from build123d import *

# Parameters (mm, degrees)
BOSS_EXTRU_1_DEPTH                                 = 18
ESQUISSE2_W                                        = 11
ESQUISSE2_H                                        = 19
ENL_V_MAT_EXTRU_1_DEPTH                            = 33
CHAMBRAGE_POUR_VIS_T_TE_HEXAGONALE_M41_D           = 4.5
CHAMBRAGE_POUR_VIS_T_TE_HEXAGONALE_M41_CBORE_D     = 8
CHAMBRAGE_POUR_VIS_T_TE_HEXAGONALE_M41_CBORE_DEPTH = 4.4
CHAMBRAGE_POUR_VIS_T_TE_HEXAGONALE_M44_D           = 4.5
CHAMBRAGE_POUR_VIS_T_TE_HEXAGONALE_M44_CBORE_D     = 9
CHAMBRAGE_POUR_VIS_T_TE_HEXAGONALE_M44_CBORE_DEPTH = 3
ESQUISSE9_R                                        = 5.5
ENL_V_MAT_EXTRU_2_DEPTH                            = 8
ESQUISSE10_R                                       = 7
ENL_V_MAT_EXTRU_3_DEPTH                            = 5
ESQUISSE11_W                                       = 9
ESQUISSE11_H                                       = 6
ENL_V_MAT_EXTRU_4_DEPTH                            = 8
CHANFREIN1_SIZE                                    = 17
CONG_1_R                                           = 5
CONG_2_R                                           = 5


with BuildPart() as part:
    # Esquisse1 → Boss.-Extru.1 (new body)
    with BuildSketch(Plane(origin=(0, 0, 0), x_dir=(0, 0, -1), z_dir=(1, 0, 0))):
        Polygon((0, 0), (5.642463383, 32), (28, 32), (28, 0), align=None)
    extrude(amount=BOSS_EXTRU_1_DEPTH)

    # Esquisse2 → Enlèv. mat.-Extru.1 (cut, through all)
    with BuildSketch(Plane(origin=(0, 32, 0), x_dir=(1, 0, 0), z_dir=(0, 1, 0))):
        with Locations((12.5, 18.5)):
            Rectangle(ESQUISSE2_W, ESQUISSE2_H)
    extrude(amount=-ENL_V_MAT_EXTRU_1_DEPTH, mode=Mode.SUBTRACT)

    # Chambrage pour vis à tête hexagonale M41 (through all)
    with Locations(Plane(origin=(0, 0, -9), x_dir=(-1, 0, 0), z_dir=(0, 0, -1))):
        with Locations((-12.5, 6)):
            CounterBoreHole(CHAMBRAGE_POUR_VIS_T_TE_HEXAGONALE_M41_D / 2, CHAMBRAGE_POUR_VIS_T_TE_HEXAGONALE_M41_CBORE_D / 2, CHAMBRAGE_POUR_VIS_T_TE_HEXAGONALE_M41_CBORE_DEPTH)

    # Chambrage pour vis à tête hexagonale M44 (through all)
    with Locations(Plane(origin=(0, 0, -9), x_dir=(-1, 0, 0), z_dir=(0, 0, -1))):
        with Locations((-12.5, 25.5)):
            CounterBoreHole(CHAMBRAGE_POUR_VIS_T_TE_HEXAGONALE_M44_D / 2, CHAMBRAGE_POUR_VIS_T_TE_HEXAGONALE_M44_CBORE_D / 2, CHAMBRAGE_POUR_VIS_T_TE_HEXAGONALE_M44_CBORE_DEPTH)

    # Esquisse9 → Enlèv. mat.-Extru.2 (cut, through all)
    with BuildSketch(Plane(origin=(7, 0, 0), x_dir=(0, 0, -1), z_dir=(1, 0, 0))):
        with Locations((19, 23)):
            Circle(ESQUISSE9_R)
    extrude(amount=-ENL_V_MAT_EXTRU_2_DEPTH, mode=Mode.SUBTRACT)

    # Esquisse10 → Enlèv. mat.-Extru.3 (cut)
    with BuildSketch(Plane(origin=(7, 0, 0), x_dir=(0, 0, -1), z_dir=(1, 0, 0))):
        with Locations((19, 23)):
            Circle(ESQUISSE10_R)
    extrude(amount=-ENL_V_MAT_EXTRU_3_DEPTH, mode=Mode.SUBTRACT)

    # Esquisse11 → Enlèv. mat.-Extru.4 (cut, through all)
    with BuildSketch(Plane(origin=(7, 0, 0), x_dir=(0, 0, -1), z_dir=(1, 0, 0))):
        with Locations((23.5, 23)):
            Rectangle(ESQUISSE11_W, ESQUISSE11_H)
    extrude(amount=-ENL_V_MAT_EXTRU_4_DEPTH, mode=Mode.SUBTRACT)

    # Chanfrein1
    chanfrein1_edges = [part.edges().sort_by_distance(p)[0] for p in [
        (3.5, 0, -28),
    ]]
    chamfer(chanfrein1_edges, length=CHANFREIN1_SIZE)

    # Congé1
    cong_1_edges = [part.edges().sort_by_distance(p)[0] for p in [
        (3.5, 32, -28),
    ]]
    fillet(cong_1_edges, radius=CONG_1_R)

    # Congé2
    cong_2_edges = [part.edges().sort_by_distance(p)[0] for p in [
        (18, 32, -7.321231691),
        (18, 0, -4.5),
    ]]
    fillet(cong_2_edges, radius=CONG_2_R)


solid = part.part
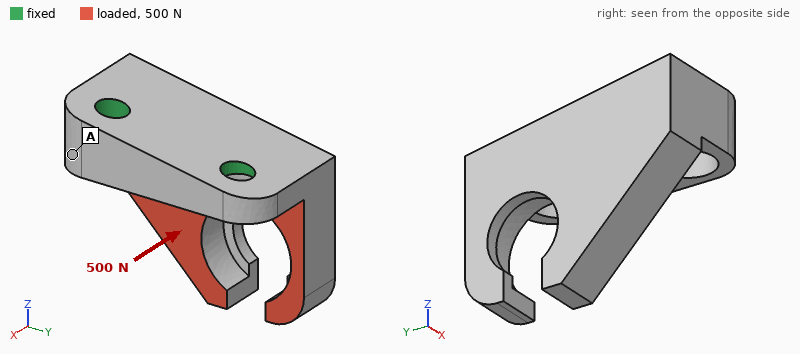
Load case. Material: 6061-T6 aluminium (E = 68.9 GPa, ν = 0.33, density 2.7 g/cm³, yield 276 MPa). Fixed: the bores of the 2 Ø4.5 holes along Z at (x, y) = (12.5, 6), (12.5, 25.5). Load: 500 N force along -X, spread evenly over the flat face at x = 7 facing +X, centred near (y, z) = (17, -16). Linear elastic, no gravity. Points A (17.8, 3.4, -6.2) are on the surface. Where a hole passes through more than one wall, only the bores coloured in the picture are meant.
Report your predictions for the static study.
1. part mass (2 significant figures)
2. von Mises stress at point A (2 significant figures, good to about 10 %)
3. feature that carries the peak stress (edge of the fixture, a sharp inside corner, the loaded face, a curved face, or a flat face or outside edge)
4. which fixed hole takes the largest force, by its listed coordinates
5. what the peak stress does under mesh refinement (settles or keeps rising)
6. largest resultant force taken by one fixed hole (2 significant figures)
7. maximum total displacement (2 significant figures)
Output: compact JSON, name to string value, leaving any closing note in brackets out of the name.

{"part mass": "14 g", "von Mises stress at point A": "14 MPa", "feature that carries the peak stress": "edge of the fixture", "which fixed hole takes the largest force, by its listed coordinates": "(12.5, 25.5)", "what the peak stress does under mesh refinement": "keeps rising", "largest resultant force taken by one fixed hole": "290 N", "maximum total displacement": "0.10 mm"}
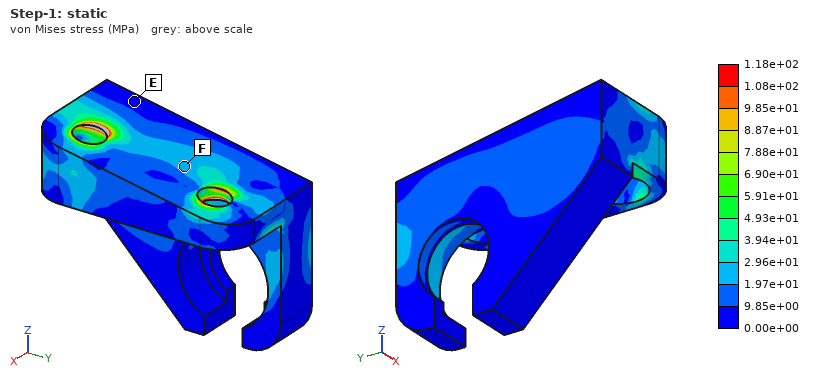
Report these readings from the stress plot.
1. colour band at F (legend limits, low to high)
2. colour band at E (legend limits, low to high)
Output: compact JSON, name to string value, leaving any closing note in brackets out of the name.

{"colour band at F": "1.97e+01 to 2.96e+01 MPa", "colour band at E": "0.00e+00 to 9.85e+00 MPa"}
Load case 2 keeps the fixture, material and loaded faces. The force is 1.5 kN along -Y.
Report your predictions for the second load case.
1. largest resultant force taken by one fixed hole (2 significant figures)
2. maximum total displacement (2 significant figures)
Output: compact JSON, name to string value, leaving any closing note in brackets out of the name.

{"largest resultant force taken by one fixed hole": "1.2 kN", "maximum total displacement": "0.19 mm"}
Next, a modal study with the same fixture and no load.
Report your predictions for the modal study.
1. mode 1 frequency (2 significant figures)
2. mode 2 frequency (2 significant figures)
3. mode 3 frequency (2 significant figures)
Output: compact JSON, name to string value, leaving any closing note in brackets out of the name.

{"mode 1 frequency": "5600 Hz", "mode 2 frequency": "8500 Hz", "mode 3 frequency": "11 kHz"}
